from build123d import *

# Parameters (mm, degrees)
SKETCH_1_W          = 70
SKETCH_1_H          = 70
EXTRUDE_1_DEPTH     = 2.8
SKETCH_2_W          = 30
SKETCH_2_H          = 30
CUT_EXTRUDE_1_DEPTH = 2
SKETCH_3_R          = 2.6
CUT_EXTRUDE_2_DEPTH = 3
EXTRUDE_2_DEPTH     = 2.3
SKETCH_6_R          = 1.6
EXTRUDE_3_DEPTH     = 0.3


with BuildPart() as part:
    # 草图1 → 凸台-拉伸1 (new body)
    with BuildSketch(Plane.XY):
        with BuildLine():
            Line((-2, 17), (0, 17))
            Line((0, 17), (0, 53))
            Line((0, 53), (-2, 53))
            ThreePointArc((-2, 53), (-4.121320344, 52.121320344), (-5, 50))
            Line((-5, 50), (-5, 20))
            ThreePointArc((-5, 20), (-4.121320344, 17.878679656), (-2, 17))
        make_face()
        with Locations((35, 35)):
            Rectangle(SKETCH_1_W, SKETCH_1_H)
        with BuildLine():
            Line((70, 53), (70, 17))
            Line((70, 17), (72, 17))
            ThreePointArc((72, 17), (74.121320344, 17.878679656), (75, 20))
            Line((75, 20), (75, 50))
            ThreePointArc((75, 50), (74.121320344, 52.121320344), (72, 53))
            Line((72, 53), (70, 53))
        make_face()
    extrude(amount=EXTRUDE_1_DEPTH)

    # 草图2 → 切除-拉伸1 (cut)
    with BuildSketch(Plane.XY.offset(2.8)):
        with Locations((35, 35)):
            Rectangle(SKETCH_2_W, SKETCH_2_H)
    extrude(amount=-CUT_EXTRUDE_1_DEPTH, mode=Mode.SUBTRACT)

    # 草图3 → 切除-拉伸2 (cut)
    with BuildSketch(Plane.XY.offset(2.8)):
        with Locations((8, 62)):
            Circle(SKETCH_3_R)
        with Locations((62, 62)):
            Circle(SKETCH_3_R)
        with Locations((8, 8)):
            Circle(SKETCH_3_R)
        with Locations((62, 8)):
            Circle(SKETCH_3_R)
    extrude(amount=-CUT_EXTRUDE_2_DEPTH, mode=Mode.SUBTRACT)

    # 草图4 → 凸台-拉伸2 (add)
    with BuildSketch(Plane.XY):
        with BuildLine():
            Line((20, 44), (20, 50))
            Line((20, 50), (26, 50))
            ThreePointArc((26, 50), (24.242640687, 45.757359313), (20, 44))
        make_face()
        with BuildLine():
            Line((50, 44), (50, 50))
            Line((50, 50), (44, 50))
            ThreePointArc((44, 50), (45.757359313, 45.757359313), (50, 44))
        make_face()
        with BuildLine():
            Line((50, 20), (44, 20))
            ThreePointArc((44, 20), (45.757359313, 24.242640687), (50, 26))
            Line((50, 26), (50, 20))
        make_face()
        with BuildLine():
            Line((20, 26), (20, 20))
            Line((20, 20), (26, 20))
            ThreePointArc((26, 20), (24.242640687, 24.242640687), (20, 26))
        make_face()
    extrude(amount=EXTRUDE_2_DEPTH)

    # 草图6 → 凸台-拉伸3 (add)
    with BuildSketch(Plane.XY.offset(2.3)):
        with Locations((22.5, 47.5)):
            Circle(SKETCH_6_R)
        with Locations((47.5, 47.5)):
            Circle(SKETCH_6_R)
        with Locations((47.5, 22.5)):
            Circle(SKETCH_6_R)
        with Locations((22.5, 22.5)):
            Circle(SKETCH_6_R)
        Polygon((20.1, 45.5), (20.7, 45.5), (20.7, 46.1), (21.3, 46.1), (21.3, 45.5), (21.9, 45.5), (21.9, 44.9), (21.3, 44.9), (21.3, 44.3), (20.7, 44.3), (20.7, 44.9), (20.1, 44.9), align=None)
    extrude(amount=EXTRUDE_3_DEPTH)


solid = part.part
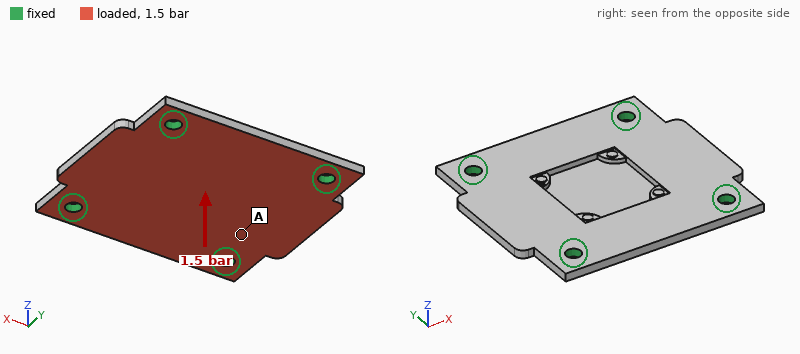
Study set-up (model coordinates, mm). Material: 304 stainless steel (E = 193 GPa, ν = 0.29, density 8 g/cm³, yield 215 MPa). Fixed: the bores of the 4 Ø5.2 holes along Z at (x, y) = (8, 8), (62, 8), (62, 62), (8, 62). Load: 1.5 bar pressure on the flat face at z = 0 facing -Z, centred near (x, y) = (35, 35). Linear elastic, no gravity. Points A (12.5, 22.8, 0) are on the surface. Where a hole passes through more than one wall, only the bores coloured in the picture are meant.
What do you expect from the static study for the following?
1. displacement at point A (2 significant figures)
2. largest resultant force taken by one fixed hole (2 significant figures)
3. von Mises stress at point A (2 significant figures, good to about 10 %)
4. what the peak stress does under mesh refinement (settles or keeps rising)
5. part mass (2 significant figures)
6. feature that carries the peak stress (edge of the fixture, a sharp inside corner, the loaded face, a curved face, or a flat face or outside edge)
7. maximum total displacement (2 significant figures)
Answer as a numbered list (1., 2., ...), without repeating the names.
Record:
1. 10 µm
2. 220 N
3. 12 MPa
4. keeps rising
5. 100 g
6. edge of the fixture
7. 42 µm
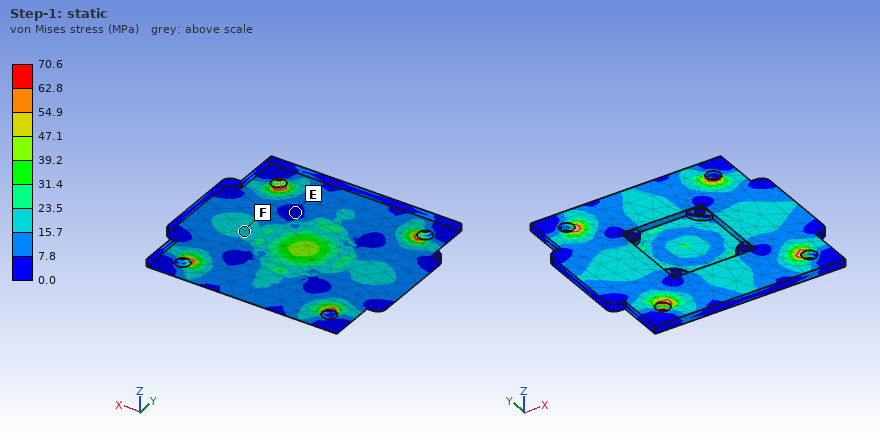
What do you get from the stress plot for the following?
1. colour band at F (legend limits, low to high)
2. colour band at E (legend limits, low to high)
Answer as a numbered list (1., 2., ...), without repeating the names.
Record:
1. 15.7 to 23.5 MPa
2. 0.0 to 7.8 MPa
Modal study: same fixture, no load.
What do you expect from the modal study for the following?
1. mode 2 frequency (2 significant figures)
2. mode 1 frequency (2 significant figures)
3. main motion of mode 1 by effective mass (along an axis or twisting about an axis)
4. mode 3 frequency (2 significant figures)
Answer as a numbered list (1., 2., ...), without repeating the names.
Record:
1. 4900 Hz
2. 4000 Hz
3. along Z
4. 4900 Hz
